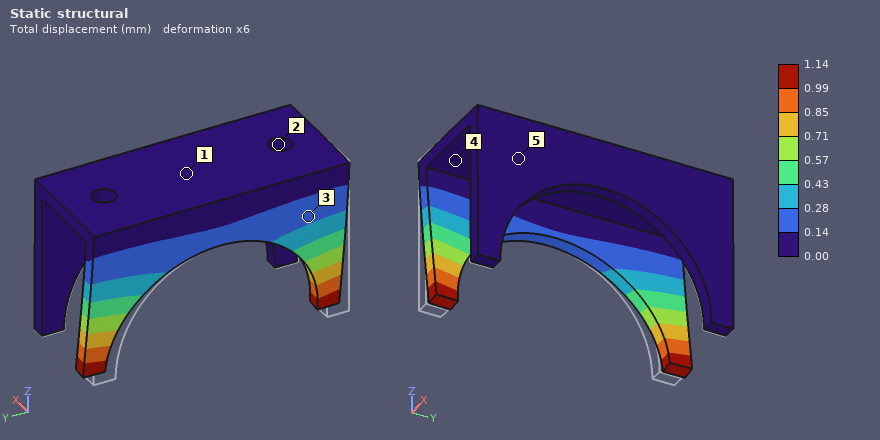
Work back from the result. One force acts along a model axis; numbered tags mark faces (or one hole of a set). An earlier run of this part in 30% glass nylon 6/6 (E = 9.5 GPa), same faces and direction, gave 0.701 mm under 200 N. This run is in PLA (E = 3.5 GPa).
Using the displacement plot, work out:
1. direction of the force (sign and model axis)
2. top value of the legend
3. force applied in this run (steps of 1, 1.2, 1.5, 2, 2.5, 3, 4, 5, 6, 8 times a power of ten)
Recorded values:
+X
1.14 mm
120 N
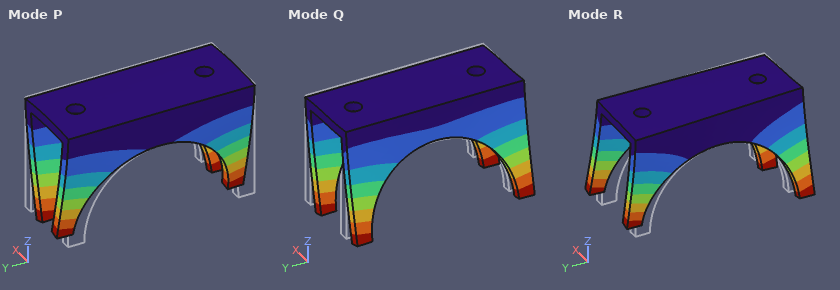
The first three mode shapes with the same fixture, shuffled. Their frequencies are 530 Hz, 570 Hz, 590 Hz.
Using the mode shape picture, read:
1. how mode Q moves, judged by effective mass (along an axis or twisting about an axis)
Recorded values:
along X
